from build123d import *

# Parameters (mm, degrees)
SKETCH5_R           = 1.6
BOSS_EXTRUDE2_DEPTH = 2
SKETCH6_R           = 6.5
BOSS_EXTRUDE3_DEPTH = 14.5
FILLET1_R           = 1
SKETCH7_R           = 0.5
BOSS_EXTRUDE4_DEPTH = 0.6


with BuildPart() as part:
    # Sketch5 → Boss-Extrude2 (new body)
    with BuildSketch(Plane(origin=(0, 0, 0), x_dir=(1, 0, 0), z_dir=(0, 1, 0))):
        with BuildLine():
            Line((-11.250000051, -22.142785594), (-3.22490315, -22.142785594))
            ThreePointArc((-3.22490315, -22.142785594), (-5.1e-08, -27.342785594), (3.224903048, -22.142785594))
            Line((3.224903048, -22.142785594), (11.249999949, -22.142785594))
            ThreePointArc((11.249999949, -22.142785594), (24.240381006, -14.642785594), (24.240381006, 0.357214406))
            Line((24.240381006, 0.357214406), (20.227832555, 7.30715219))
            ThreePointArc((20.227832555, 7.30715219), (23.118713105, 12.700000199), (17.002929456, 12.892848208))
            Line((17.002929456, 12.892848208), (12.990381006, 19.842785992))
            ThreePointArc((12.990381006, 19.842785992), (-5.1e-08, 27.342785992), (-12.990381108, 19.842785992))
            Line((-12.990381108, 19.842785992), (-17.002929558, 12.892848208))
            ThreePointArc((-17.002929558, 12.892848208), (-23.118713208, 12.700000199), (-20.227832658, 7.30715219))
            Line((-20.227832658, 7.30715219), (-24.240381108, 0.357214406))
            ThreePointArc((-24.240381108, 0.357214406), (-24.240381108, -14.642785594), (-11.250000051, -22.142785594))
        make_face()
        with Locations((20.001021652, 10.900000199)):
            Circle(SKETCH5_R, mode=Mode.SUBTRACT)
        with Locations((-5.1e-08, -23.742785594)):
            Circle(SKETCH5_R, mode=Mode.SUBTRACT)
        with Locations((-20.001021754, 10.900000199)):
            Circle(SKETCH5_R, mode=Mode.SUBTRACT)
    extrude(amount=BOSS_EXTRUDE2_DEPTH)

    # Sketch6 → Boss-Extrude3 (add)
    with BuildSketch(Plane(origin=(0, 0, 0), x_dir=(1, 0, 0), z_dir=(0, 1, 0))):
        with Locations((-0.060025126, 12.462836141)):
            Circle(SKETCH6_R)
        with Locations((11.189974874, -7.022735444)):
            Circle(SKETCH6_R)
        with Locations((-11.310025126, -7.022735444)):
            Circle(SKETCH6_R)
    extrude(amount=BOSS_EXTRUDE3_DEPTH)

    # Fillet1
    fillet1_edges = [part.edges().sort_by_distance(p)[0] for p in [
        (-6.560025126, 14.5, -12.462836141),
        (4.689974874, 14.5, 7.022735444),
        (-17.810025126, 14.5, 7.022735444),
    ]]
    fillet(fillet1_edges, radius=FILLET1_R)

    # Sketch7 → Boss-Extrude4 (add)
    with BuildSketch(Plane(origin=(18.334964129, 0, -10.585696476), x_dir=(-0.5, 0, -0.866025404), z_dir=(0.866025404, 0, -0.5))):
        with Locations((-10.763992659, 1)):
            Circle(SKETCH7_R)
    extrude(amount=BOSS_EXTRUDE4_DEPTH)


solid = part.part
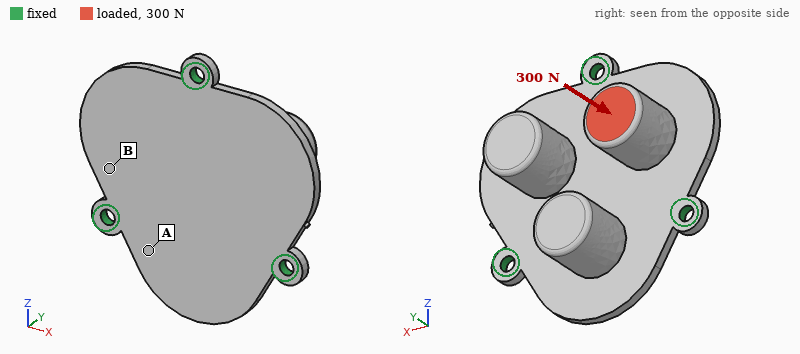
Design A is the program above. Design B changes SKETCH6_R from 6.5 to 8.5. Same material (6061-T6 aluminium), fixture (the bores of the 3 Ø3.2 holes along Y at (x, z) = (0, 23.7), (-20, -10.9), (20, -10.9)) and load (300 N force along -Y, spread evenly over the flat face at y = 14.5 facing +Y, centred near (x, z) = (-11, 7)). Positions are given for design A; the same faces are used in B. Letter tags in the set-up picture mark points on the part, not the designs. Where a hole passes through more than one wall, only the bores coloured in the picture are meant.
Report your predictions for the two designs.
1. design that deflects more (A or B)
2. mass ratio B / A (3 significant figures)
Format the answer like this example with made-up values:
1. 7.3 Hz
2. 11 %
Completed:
1. A
2. 1.39
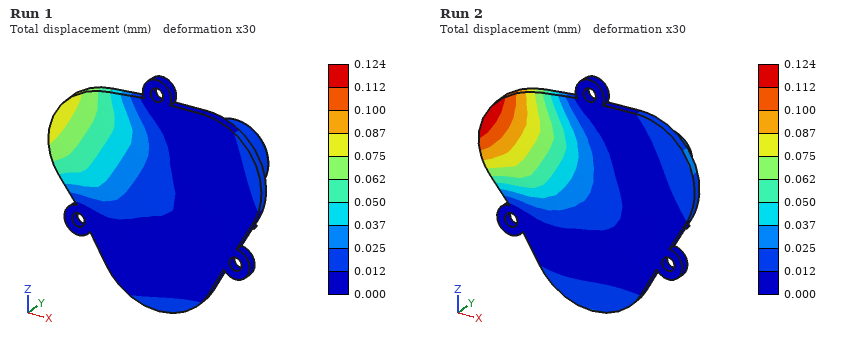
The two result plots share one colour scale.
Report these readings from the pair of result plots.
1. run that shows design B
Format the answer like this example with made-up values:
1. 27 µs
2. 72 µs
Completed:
1. Run 1
